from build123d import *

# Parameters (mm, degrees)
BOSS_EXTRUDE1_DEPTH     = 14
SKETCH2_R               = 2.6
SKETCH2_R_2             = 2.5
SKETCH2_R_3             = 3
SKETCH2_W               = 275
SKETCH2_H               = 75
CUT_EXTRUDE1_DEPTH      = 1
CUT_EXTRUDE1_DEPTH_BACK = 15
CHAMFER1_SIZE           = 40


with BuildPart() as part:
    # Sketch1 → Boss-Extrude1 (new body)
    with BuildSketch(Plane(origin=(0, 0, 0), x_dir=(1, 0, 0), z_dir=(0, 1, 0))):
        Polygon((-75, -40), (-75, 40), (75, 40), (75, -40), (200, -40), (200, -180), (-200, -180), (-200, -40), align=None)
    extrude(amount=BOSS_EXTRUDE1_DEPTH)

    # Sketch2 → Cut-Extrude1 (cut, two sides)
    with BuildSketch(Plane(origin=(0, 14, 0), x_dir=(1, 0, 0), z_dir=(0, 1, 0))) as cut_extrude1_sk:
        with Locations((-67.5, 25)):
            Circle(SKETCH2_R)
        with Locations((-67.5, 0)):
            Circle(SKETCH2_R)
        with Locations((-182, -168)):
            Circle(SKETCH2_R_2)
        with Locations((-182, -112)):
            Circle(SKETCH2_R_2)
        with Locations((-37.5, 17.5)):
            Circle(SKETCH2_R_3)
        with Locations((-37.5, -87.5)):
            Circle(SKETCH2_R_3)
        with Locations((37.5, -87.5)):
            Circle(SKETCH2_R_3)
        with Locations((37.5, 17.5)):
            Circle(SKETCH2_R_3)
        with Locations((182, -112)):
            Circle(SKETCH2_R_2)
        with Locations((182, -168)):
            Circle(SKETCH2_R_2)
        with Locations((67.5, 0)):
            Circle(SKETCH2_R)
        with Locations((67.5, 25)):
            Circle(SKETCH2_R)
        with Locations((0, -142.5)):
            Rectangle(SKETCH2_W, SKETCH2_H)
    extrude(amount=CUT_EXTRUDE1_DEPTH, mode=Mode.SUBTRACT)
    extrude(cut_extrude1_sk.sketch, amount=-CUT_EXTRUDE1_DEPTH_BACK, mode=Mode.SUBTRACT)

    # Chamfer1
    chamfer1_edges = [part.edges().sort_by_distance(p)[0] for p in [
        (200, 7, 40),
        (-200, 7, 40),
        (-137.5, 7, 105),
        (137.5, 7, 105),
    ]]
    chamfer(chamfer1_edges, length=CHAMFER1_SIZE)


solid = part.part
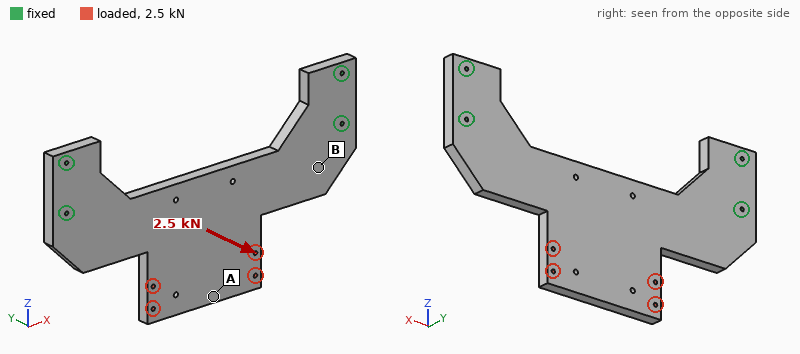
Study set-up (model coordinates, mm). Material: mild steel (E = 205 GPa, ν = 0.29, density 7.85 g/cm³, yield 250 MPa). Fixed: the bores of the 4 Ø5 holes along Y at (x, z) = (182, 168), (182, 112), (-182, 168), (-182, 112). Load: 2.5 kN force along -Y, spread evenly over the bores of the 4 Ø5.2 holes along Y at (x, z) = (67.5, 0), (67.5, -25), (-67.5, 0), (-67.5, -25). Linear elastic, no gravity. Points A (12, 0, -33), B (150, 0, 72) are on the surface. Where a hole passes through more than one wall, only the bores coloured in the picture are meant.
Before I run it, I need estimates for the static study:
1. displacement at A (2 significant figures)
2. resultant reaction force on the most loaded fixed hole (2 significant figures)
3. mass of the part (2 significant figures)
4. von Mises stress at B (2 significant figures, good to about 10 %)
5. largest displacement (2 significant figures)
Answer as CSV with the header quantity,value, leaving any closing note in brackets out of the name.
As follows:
quantity,value
displacement at A,0.67 mm
resultant reaction force on the most loaded fixed hole,3.0 kN
mass of the part,5.2 kg
von Mises stress at B,36 MPa
largest displacement,0.70 mm
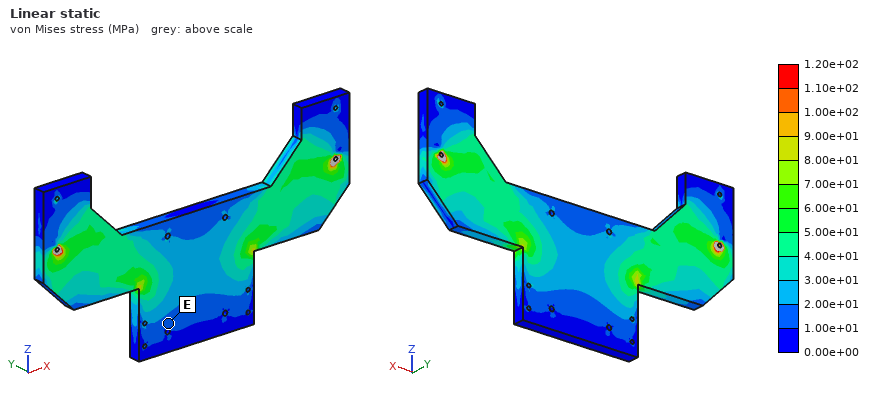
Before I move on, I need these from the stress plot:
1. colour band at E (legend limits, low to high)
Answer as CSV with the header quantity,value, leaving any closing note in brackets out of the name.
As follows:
quantity,value
colour band at E,1.00e+01 to 2.00e+01 MPa
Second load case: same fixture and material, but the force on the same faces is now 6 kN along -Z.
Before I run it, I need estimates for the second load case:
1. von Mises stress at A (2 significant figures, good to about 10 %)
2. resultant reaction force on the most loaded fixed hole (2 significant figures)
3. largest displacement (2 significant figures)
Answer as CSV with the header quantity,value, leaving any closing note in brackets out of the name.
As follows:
quantity,value
von Mises stress at A,2.5 MPa
resultant reaction force on the most loaded fixed hole,2.8 kN
largest displacement,12 µm
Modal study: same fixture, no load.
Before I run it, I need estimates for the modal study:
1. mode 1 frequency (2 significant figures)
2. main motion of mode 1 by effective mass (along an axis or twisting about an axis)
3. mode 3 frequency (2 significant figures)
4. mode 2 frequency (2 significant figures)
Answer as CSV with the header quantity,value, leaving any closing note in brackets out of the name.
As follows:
quantity,value
mode 1 frequency,280 Hz
main motion of mode 1 by effective mass,along Y
mode 3 frequency,960 Hz
mode 2 frequency,810 Hz
